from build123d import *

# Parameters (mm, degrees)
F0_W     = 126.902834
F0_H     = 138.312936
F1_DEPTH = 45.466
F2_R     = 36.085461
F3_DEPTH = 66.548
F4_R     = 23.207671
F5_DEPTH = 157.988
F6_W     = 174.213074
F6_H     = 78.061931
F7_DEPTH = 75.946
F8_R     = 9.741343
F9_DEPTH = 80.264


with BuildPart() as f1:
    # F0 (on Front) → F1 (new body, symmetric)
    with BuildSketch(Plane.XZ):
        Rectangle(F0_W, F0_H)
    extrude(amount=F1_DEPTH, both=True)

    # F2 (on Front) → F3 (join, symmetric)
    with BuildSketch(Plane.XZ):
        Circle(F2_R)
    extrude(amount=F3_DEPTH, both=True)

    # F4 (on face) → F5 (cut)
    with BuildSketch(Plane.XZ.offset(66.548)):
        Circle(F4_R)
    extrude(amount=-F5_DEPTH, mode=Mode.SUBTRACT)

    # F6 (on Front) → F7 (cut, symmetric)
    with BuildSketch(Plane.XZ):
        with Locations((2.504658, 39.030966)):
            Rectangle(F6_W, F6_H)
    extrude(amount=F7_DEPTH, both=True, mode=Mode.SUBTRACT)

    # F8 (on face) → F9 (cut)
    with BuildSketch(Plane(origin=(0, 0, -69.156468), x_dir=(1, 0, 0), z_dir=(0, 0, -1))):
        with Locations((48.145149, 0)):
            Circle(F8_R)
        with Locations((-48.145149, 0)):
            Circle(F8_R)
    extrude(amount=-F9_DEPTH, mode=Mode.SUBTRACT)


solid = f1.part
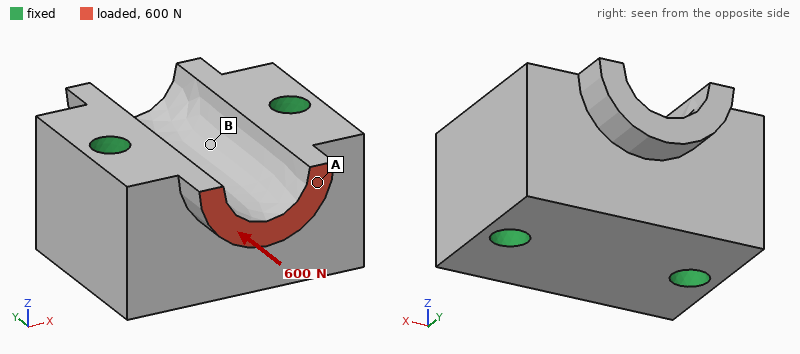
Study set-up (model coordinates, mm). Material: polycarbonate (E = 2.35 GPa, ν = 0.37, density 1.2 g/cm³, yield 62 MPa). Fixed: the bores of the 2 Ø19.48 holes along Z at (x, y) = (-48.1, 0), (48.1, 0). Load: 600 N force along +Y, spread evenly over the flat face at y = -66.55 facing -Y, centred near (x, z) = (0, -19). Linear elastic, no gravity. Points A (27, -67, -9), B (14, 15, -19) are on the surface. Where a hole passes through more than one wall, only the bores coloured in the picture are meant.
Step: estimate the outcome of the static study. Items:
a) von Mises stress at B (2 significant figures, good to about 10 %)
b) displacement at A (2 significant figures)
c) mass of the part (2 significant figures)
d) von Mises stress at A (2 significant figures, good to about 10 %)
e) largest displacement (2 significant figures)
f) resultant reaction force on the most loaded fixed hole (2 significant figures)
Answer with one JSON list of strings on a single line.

["0.069 MPa", "13 µm", "880 g", "0.50 MPa", "15 µm", "320 N"]
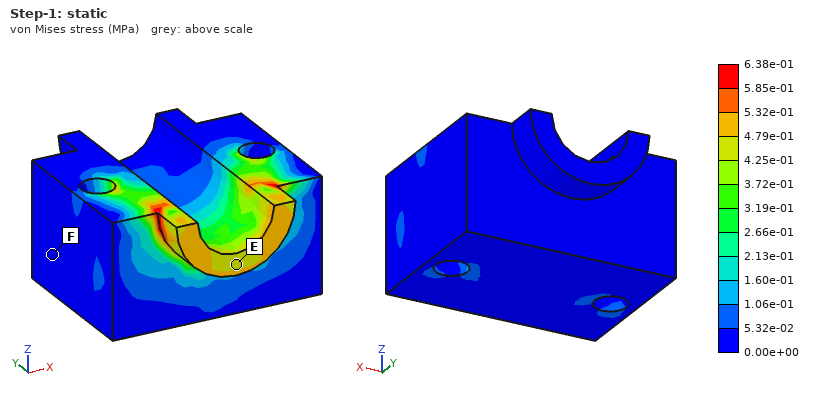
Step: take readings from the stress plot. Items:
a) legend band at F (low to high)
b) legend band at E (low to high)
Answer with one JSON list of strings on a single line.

["0.00e+00 to 5.32e-02 MPa", "4.25e-01 to 4.79e-01 MPa"]
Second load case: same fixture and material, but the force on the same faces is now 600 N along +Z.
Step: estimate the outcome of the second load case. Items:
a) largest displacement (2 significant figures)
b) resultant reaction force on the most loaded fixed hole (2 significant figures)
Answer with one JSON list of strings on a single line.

["87 µm", "300 N"]
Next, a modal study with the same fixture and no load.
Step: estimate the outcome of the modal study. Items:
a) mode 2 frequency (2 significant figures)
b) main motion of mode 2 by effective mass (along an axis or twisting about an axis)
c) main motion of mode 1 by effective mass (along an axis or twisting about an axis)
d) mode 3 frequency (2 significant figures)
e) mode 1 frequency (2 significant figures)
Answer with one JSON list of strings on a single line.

["2900 Hz", "along Z", "twisting about X", "3200 Hz", "2800 Hz"]
